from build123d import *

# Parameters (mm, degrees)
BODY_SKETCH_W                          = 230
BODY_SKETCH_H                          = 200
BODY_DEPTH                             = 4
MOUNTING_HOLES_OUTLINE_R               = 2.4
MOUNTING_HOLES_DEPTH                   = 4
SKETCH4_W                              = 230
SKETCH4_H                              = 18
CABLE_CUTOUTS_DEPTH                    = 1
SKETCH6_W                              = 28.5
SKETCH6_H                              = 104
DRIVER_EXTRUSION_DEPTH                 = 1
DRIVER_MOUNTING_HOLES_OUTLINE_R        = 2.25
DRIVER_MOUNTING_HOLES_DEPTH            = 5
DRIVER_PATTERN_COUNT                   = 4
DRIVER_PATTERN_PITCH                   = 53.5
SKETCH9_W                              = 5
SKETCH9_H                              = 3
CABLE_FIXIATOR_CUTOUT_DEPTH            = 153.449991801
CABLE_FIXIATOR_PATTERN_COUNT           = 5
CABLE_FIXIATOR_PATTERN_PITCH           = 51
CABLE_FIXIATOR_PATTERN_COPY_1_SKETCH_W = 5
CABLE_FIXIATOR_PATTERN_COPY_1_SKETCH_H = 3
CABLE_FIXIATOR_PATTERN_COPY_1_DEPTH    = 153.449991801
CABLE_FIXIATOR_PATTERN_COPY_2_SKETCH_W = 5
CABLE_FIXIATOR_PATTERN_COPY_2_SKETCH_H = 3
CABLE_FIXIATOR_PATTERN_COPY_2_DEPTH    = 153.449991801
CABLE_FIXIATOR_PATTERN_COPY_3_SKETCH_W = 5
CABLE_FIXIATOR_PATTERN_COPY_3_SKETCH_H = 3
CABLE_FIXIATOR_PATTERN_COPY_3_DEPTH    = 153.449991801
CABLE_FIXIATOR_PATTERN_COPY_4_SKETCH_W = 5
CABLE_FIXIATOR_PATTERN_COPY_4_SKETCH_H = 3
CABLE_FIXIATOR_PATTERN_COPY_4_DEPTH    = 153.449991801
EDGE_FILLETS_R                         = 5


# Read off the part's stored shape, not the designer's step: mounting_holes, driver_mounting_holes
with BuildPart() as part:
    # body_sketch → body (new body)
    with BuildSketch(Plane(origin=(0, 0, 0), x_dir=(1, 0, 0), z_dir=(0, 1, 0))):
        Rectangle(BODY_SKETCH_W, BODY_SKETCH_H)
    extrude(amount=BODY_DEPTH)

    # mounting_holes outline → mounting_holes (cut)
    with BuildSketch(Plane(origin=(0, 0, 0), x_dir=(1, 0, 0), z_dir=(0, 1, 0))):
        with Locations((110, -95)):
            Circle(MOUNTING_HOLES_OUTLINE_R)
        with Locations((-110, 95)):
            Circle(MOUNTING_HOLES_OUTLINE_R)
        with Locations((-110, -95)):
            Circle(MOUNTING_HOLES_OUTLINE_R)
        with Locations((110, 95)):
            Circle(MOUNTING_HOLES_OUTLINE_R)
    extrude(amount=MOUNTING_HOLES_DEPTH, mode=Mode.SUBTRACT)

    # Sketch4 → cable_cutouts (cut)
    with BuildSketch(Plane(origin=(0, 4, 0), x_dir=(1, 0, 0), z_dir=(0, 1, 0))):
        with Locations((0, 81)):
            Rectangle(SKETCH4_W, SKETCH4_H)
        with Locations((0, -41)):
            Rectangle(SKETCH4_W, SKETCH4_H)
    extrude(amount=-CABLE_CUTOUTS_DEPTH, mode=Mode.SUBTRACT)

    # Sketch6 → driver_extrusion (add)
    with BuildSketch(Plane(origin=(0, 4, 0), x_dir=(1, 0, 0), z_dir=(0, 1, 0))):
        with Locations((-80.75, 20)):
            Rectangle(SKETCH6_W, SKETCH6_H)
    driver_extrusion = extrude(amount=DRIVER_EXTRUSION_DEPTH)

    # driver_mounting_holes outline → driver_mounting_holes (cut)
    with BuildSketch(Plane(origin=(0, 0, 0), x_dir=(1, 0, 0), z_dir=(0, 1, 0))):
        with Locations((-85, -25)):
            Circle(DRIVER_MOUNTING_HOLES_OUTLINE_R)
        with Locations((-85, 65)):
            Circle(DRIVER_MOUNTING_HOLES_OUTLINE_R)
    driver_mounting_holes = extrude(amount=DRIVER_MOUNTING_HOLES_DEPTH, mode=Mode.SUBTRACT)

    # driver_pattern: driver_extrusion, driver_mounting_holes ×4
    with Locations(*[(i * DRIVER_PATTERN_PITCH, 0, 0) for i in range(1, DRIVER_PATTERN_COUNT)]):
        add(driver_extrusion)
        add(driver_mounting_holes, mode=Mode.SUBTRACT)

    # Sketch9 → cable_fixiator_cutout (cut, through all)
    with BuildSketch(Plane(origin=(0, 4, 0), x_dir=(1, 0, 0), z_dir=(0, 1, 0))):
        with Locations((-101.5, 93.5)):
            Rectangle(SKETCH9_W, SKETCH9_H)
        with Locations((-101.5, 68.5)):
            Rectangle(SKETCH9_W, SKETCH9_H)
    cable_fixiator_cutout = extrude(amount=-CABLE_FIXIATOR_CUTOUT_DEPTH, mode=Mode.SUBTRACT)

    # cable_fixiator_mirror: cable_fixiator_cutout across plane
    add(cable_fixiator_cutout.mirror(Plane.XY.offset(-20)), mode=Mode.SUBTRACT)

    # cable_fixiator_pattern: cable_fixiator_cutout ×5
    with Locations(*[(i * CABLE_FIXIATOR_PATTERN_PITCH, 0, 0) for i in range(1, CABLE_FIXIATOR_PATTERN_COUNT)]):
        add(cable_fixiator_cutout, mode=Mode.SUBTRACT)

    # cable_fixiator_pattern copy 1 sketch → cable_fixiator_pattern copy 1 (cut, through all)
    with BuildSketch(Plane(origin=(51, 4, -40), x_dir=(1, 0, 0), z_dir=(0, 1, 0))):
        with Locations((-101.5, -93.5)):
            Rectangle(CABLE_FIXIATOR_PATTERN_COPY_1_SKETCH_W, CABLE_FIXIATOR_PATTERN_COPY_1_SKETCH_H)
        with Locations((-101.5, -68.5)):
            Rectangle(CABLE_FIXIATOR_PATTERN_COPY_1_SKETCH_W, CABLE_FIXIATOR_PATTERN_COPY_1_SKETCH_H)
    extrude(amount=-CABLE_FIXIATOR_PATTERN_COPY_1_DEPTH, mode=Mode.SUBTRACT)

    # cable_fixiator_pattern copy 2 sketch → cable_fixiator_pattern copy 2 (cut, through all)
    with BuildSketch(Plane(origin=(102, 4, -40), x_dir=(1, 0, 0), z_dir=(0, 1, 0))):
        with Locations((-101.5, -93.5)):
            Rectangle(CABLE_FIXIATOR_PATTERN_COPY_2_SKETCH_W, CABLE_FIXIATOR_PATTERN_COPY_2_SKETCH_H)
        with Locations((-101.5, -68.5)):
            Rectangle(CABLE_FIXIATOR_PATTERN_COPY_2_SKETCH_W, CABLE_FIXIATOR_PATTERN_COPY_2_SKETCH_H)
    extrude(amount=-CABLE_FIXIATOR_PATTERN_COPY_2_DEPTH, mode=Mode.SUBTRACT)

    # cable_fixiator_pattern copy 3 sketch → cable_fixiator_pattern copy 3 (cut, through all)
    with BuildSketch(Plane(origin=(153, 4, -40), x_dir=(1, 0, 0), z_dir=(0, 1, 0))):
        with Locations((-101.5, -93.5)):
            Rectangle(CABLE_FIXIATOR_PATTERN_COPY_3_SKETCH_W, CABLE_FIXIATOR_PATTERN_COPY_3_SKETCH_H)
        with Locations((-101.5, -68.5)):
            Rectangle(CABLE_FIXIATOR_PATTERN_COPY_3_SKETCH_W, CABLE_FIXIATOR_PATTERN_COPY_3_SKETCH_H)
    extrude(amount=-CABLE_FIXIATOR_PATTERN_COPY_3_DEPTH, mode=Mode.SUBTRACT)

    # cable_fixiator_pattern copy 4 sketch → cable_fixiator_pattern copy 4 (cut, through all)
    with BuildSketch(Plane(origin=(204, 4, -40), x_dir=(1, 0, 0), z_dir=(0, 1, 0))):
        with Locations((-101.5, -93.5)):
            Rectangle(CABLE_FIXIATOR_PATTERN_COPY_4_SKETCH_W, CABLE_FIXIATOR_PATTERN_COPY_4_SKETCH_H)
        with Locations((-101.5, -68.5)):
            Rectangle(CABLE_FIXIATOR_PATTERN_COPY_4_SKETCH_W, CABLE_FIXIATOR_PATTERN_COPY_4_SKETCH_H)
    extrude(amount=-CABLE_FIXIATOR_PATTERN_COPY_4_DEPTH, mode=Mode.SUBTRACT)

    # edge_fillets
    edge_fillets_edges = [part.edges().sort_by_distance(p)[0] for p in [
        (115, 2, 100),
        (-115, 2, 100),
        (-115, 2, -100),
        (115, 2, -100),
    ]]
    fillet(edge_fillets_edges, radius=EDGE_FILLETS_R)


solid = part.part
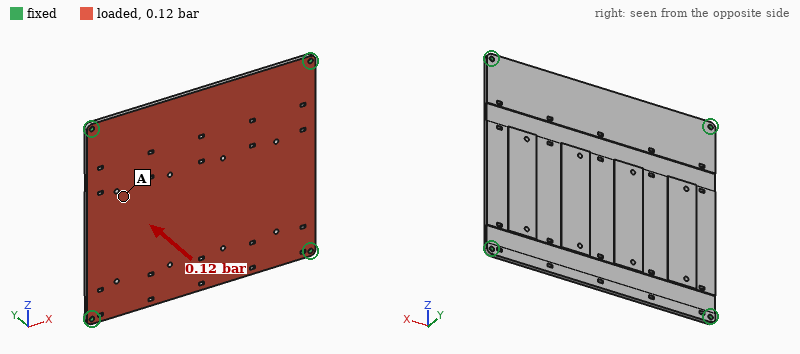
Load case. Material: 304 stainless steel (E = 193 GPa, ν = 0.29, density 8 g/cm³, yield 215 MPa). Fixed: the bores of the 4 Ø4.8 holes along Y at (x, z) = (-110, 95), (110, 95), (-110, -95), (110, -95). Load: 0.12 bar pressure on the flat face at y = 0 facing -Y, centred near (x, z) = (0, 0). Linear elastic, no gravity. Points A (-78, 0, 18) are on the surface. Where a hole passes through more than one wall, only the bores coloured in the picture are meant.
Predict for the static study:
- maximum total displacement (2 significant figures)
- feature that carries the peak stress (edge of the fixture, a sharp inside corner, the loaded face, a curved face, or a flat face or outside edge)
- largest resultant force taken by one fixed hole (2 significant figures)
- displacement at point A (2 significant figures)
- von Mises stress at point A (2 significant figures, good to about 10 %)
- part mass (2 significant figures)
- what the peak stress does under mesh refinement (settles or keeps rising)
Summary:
0.20 mm
edge of the fixture
160 N
0.13 mm
8.0 MPa
1.5 kg
keeps rising
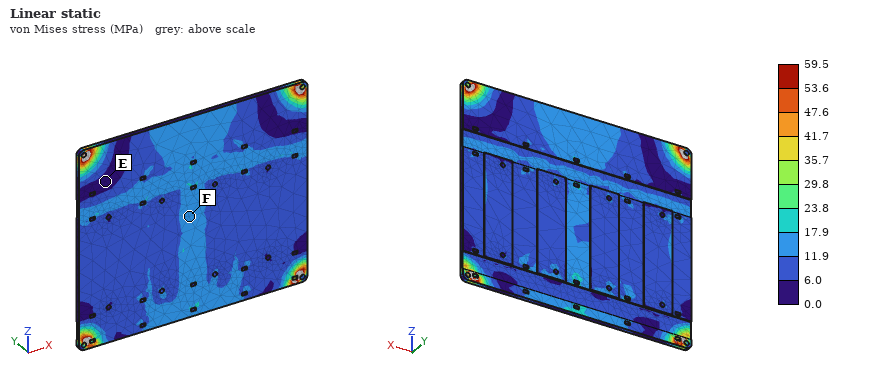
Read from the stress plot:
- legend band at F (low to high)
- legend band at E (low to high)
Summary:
11.9 to 17.9 MPa
0.0 to 6.0 MPa
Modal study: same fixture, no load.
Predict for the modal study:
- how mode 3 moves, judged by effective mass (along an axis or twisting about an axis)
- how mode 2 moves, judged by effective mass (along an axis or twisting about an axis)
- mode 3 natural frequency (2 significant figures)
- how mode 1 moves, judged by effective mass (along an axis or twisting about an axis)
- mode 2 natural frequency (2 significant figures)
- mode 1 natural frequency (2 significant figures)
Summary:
twisting about Z
twisting about X
510 Hz
along Y
470 Hz
250 Hz
